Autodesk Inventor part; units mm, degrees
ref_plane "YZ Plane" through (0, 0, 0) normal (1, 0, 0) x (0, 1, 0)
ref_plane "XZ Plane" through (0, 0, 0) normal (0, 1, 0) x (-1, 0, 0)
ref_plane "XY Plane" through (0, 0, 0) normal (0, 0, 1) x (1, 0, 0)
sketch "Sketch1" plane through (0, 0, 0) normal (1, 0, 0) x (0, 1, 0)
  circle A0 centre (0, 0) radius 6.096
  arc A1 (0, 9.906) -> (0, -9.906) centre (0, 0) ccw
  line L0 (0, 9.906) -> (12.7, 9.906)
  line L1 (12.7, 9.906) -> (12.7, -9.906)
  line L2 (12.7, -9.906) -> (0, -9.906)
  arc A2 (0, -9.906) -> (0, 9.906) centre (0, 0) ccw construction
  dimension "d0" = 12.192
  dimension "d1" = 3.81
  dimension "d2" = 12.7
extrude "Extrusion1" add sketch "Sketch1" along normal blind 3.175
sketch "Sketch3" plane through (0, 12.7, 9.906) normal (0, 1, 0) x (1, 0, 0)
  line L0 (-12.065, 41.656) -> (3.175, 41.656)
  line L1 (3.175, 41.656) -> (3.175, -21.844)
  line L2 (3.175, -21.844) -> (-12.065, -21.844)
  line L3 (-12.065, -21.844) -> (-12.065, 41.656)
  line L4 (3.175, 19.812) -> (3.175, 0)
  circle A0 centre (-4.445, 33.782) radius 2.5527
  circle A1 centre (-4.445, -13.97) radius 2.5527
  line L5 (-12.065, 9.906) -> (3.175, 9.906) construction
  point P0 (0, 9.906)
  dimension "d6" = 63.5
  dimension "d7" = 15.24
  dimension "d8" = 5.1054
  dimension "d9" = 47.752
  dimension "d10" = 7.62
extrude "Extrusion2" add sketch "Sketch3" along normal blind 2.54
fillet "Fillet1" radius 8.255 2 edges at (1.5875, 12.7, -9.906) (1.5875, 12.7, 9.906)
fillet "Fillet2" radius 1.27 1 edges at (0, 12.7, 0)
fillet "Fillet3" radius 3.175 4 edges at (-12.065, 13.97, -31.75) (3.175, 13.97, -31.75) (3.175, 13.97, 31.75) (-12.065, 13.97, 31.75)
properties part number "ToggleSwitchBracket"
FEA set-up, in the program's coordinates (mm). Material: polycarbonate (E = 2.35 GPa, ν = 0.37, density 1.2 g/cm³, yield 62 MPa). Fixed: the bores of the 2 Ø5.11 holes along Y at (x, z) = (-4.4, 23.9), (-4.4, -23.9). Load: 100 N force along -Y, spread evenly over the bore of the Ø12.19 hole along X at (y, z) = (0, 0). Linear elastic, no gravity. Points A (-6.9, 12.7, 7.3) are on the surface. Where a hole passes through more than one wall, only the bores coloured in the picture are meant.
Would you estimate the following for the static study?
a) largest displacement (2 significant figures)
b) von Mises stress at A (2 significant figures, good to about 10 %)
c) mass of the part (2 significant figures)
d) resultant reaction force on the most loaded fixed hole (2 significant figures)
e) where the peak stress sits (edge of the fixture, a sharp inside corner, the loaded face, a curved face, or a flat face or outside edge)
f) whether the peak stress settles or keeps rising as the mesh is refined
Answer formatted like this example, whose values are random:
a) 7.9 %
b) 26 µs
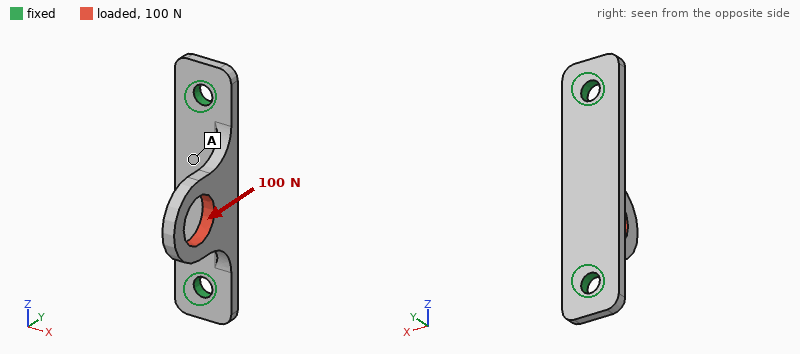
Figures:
a) 0.83 mm
b) 3.0 MPa
c) 4.0 g
d) 65 N
e) edge of the fixture
f) keeps rising
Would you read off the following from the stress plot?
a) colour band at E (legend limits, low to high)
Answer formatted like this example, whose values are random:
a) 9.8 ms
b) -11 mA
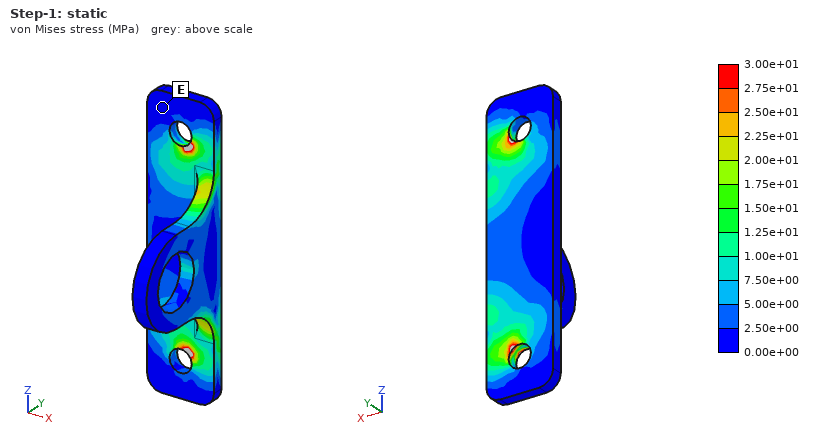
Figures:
a) 0.00e+00 to 2.50e+00 MPa
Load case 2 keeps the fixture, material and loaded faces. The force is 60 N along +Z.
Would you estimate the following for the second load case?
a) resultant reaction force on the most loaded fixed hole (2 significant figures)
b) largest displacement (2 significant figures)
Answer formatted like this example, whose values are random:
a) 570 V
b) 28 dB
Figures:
a) 38 N
b) 0.24 mm
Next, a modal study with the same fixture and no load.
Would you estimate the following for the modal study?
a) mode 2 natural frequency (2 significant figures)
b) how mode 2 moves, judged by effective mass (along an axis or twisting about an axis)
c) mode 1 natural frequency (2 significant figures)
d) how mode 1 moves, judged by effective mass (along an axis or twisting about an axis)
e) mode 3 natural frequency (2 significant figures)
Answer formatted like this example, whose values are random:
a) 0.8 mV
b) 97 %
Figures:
a) 2100 Hz
b) along Y
c) 980 Hz
d) along X
e) 2900 Hz
